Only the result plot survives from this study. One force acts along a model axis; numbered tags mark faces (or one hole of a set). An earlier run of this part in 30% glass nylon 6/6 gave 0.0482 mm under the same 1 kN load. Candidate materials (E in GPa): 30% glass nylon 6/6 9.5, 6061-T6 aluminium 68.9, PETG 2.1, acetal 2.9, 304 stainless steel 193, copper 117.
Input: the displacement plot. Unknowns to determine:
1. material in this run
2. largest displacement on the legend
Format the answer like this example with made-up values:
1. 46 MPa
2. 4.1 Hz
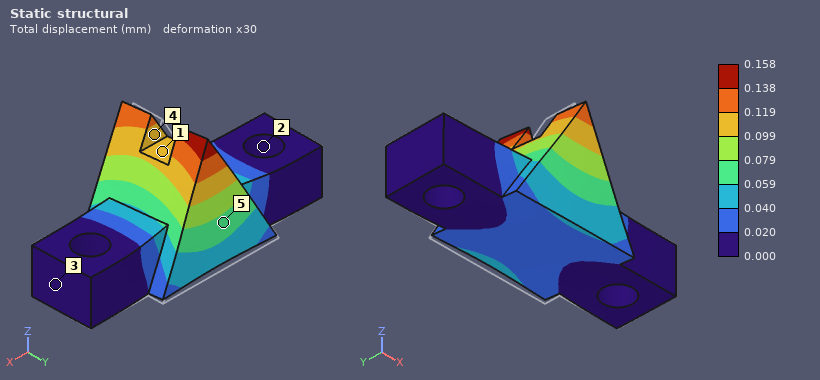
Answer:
1. acetal
2. 0.158 mm
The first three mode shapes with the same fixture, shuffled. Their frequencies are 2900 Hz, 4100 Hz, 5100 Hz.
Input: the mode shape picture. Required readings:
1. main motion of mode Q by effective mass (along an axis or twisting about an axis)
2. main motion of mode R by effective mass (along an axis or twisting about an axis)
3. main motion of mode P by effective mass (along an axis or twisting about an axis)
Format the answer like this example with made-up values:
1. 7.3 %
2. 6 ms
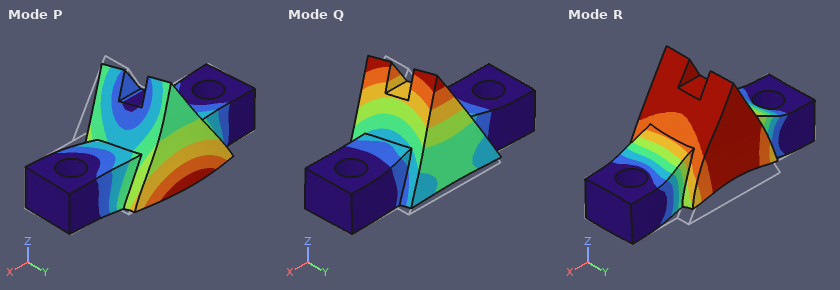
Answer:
1. along Y
2. along Z
3. along Y
